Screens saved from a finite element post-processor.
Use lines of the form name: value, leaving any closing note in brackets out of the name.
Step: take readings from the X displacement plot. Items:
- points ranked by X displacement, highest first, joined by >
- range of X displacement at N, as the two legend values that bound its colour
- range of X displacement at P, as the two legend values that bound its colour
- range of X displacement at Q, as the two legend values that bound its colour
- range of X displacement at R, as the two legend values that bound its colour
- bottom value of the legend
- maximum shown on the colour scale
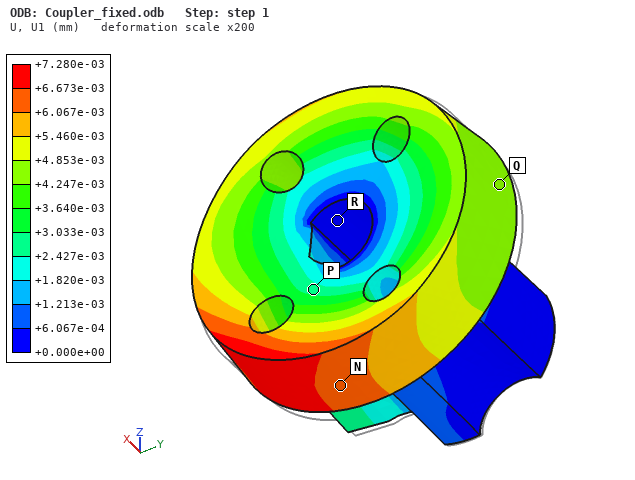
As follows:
points ranked by X displacement, highest first, joined by >: N > Q > P > R
range of X displacement at N, as the two legend values that bound its colour: +6.067e-03 to +6.673e-03 mm
range of X displacement at P, as the two legend values that bound its colour: +2.427e-03 to +3.033e-03 mm
range of X displacement at Q, as the two legend values that bound its colour: +4.247e-03 to +4.853e-03 mm
range of X displacement at R, as the two legend values that bound its colour: +0.000e+00 to +6.067e-04 mm
bottom value of the legend: +0.000e+00 mm
maximum shown on the colour scale: +7.280e-03 mm
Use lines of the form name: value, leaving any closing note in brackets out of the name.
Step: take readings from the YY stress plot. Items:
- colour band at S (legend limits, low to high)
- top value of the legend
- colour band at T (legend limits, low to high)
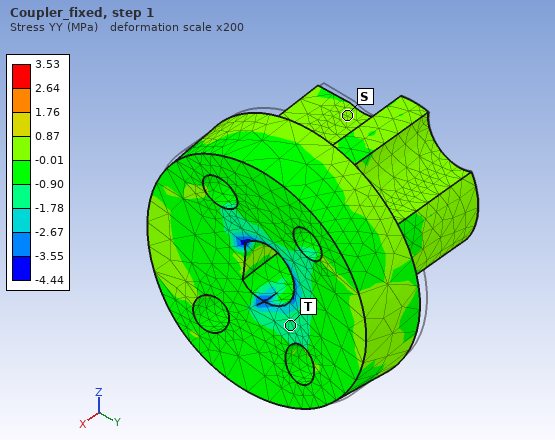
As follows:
colour band at S: -0.01 to 0.87 MPa
top value of the legend: 3.53 MPa
colour band at T: -1.78 to -0.90 MPa
